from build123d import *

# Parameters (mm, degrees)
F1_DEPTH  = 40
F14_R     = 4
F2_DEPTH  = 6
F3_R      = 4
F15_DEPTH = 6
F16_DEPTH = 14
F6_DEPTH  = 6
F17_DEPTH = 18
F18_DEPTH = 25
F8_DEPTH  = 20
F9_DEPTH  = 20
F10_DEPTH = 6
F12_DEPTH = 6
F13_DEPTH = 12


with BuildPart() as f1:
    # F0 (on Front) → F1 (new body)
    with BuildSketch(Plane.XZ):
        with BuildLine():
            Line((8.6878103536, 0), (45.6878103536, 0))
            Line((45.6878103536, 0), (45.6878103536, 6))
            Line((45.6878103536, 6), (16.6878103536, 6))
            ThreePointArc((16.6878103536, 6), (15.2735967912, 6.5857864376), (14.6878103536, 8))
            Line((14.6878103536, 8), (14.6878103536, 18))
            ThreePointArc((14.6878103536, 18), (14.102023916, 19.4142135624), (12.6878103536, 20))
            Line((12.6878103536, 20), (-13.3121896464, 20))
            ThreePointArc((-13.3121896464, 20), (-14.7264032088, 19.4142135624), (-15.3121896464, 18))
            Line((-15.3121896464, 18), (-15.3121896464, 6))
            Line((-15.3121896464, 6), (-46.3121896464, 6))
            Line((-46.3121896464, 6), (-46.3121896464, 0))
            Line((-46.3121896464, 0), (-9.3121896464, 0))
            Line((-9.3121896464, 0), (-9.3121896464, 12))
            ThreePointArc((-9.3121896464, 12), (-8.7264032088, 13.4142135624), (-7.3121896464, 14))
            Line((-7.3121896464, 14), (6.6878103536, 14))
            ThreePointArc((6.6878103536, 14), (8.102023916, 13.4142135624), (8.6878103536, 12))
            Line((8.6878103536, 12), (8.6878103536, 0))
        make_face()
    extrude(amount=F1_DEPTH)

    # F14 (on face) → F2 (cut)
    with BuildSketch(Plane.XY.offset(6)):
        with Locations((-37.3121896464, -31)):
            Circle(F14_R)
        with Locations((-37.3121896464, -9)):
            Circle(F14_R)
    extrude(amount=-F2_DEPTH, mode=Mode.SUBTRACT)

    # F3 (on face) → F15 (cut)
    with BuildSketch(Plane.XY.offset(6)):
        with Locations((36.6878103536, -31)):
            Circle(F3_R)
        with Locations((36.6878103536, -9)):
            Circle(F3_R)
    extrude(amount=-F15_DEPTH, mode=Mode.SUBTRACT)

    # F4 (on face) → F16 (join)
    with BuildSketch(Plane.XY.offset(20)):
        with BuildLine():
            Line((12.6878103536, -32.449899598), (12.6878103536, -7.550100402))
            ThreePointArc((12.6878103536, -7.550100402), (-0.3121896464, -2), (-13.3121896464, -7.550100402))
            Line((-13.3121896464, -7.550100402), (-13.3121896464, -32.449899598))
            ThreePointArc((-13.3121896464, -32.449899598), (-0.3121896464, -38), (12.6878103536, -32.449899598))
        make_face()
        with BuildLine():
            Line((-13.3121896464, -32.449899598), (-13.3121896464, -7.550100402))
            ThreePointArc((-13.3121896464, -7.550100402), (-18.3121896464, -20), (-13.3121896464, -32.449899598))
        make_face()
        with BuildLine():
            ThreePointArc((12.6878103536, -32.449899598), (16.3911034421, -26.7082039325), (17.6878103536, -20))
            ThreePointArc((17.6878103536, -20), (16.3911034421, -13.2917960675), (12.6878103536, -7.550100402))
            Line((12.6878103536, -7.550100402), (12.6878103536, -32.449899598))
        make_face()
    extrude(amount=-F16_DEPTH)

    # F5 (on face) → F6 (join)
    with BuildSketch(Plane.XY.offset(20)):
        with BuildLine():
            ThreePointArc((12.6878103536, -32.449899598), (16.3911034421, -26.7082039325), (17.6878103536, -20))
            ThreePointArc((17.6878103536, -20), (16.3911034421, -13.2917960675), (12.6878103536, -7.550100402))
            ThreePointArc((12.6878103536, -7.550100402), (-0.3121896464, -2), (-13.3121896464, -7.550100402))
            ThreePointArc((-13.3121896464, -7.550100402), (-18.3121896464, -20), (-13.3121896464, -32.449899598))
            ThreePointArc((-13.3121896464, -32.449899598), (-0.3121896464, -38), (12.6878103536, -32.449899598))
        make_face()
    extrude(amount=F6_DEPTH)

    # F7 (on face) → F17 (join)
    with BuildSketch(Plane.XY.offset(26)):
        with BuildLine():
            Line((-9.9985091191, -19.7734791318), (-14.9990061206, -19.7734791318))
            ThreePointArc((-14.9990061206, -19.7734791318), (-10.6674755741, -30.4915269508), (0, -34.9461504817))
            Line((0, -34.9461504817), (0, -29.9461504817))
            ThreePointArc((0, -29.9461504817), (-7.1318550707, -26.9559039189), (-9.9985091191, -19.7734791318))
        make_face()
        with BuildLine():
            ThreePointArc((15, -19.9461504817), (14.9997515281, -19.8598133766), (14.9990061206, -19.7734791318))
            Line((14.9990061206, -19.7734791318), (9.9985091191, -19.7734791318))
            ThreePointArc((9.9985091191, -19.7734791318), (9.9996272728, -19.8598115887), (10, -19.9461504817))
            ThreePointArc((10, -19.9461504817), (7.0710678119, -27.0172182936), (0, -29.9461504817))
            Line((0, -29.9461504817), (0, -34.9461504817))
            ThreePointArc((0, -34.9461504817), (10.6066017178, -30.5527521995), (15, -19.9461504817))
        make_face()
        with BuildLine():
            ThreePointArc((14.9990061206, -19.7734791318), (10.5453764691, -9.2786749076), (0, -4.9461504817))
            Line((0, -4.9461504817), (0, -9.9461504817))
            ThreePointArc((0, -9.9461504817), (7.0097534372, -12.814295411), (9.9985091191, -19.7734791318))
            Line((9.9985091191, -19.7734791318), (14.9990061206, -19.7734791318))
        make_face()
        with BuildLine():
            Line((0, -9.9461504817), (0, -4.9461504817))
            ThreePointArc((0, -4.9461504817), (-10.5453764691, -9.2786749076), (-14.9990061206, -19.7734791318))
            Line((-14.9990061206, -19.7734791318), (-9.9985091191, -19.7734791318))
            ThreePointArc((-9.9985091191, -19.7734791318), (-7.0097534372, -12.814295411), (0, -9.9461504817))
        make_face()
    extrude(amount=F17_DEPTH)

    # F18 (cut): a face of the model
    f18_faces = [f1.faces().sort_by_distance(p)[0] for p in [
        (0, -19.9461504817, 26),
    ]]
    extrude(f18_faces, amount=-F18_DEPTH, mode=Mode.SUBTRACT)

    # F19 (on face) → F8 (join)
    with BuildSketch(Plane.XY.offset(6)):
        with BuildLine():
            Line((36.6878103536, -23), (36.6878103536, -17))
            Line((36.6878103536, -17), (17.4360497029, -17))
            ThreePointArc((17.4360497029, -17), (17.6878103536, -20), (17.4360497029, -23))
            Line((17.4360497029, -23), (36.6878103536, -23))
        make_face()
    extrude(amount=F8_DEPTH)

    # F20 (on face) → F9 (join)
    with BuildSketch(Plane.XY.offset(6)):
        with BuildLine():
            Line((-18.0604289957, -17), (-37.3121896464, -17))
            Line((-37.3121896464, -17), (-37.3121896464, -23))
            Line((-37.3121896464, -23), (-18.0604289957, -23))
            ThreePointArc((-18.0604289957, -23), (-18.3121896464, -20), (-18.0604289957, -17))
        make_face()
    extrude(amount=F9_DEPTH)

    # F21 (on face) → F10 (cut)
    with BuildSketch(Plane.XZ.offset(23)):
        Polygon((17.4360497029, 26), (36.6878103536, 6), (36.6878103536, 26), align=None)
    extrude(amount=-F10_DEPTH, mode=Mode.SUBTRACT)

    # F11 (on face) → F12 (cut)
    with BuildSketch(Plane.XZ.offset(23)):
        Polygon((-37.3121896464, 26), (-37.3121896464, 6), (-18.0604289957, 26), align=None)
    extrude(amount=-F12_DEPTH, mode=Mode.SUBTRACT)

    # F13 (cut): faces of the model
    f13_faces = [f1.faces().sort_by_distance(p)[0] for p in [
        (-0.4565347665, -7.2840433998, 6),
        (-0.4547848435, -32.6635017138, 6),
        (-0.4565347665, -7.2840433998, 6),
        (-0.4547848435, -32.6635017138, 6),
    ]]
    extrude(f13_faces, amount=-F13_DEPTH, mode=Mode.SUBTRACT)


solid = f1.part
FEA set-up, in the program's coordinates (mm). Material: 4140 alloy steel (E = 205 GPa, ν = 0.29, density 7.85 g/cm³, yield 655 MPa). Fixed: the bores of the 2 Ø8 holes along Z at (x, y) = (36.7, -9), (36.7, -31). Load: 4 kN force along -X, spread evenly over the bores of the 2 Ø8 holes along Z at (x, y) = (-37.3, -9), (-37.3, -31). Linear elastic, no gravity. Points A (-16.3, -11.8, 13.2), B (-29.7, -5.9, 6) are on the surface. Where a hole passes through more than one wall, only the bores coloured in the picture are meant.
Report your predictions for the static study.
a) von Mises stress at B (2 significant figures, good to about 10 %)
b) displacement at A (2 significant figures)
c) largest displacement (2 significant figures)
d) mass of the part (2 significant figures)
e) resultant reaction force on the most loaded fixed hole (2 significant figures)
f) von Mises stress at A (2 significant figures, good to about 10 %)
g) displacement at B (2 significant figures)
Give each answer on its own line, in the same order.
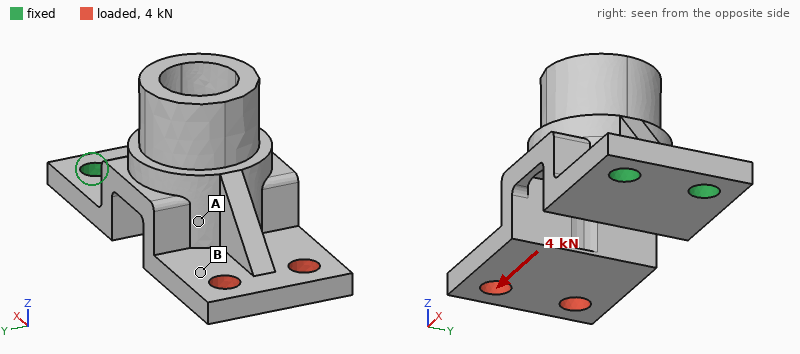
24 MPa
0.10 mm
0.29 mm
310 g
2.0 kN
87 MPa
0.19 mm
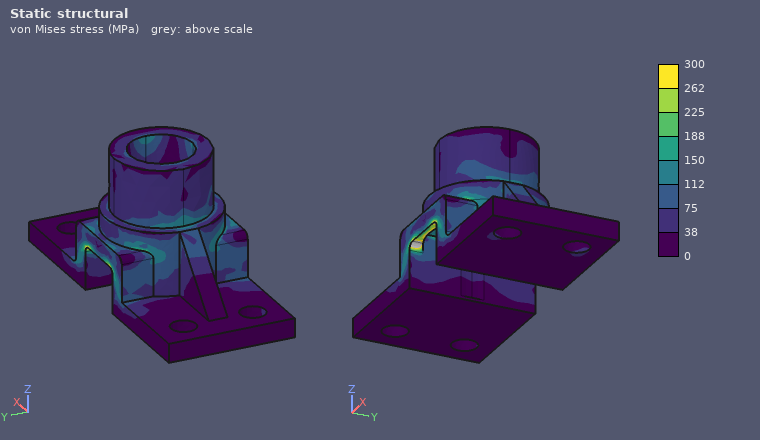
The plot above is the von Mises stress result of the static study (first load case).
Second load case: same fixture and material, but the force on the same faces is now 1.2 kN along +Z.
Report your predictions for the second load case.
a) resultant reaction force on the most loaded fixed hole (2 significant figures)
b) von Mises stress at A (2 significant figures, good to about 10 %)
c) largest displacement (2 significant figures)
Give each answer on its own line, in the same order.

710 N
33 MPa
0.50 mm
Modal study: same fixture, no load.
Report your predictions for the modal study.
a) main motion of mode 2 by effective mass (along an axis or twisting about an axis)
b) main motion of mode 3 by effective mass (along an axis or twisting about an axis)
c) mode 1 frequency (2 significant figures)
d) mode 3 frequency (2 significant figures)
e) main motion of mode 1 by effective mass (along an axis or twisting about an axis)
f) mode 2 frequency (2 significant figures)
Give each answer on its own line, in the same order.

along Y
along Y
900 Hz
2500 Hz
along Z
1800 Hz
